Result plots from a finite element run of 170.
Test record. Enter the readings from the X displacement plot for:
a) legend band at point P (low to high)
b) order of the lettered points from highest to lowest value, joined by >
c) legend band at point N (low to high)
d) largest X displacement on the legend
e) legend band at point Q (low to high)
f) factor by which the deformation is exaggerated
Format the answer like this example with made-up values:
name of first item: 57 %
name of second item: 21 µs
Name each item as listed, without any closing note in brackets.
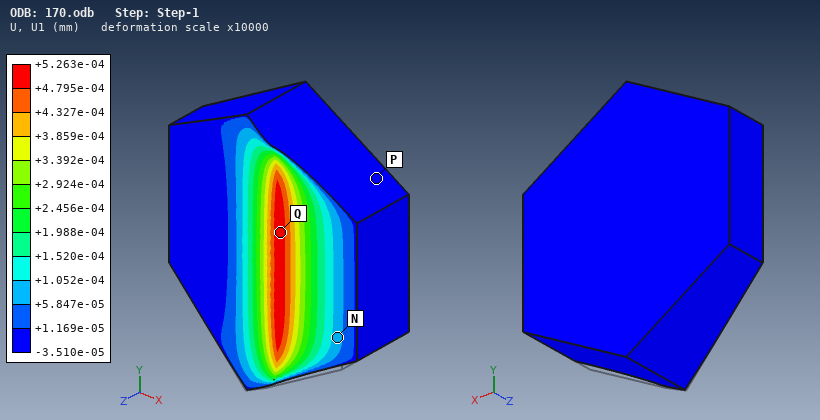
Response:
legend band at point P: -3.510e-05 to +1.169e-05 mm
order of the lettered points from highest to lowest value, joined by >: Q > N > P
legend band at point N: +5.847e-05 to +1.052e-04 mm
largest X displacement on the legend: +5.263e-04 mm
legend band at point Q: +4.795e-04 to +5.263e-04 mm
factor by which the deformation is exaggerated: 10000
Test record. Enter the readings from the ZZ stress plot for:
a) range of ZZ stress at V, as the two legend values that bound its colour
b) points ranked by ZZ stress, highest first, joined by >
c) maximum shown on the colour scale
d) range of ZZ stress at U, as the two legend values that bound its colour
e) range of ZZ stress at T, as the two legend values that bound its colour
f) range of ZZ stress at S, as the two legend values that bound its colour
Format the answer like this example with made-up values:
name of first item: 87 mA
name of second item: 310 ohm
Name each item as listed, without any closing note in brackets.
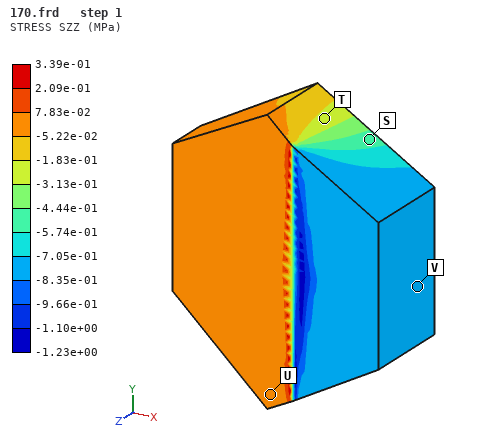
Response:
range of ZZ stress at V, as the two legend values that bound its colour: -8.35e-01 to -7.05e-01 MPa
points ranked by ZZ stress, highest first, joined by >: U > T > S > V
maximum shown on the colour scale: 3.39e-01 MPa
range of ZZ stress at U, as the two legend values that bound its colour: -5.22e-02 to 7.83e-02 MPa
range of ZZ stress at T, as the two legend values that bound its colour: -3.13e-01 to -1.83e-01 MPa
range of ZZ stress at S, as the two legend values that bound its colour: -5.74e-01 to -4.44e-01 MPa
